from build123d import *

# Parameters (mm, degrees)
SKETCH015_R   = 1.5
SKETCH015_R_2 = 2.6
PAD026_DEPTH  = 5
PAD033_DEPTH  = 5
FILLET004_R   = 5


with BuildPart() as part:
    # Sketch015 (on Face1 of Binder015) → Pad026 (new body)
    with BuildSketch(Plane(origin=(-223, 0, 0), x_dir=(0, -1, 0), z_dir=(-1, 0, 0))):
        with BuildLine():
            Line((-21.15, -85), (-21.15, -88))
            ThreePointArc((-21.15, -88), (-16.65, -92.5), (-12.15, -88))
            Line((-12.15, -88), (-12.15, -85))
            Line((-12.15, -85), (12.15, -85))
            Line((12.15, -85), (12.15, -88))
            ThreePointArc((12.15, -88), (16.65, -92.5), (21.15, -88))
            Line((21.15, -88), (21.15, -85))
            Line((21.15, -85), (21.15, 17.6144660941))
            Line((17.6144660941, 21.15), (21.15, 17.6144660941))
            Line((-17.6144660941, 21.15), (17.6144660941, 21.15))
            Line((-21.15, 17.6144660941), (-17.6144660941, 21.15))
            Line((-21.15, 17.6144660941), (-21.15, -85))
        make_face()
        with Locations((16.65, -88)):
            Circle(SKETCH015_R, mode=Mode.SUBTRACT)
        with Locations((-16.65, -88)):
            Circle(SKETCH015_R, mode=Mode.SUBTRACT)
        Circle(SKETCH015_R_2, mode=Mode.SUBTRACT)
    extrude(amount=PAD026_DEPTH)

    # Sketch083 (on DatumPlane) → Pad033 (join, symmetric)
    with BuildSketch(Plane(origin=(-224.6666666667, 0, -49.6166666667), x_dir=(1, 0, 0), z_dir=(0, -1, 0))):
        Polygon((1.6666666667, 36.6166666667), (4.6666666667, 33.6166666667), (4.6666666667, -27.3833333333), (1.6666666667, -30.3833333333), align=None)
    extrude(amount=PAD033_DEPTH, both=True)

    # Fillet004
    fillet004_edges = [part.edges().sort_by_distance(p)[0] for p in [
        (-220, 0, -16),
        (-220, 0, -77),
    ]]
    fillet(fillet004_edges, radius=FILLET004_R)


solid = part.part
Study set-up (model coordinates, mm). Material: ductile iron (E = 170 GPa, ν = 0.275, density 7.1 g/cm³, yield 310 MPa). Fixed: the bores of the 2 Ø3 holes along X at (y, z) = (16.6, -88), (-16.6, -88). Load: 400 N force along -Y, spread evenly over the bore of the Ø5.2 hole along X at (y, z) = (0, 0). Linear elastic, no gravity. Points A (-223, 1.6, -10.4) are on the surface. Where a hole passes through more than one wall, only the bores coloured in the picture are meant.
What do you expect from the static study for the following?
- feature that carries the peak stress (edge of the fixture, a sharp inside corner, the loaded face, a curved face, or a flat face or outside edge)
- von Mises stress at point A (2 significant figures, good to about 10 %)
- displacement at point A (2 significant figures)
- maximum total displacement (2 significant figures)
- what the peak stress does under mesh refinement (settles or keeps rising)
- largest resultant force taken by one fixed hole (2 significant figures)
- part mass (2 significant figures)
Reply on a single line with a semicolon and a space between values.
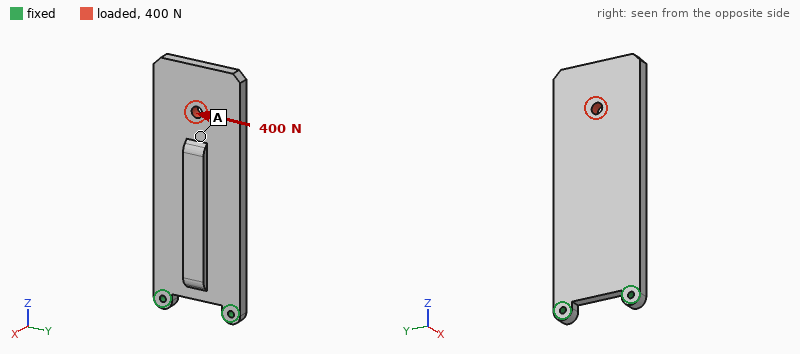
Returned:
edge of the fixture; 4.6 MPa; 17 µm; 28 µm; keeps rising; 1.0 kN; 180 g
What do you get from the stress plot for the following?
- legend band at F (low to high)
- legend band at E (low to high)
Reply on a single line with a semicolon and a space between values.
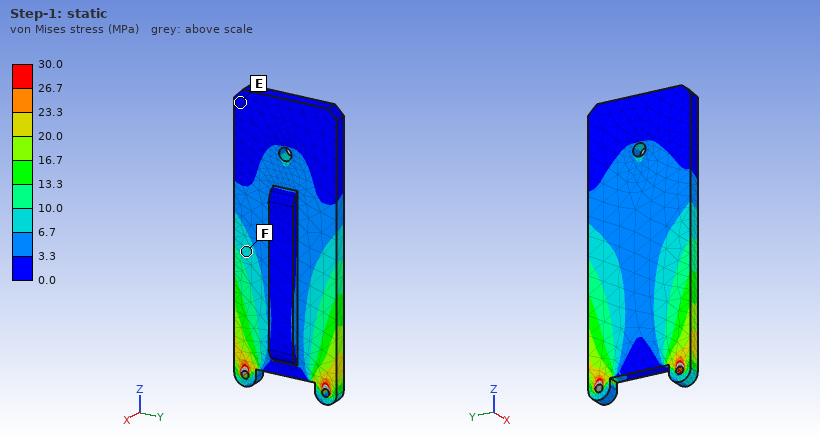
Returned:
6.7 to 10.0 MPa; 0.0 to 3.3 MPa
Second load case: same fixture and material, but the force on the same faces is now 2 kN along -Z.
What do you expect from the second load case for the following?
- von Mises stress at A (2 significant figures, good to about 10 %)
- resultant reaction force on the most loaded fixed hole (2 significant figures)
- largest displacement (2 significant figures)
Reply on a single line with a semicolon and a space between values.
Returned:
17 MPa; 1.0 kN; 23 µm
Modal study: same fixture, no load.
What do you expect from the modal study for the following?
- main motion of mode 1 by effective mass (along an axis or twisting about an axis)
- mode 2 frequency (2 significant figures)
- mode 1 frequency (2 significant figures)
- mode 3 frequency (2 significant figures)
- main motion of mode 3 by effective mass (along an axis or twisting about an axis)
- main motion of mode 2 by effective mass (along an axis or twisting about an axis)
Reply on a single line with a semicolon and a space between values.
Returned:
along X; 2000 Hz; 320 Hz; 2200 Hz; along X; twisting about Z
